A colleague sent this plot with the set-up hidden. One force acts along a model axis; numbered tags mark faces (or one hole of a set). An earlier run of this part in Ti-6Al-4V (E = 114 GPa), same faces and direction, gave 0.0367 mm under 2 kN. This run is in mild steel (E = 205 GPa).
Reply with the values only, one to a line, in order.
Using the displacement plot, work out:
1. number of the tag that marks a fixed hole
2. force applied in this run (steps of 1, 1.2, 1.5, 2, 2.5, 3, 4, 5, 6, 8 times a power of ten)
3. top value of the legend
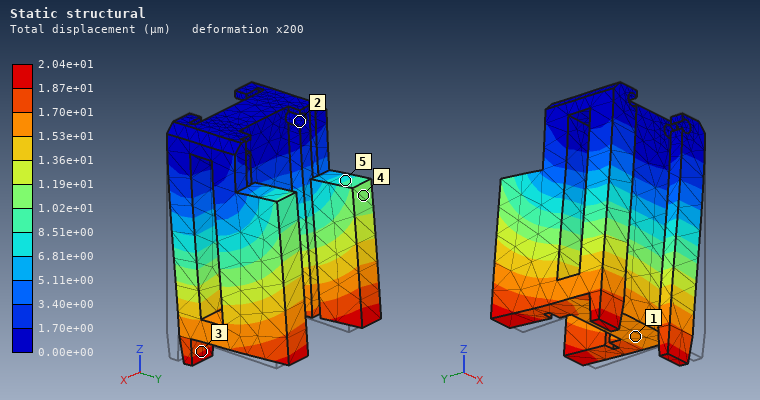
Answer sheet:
2
2 kN
2.04e+01 µm
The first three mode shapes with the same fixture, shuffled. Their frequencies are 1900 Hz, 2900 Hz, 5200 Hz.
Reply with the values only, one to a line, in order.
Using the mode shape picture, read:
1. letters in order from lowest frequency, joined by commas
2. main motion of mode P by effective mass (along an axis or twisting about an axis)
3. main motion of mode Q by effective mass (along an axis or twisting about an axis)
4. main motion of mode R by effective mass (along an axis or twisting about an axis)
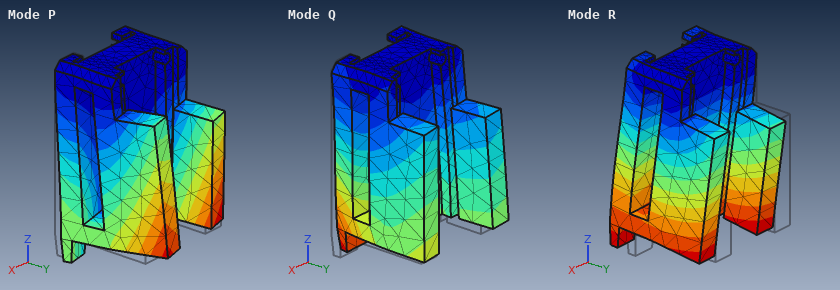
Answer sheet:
R, P, Q
along X
along X
along Y
